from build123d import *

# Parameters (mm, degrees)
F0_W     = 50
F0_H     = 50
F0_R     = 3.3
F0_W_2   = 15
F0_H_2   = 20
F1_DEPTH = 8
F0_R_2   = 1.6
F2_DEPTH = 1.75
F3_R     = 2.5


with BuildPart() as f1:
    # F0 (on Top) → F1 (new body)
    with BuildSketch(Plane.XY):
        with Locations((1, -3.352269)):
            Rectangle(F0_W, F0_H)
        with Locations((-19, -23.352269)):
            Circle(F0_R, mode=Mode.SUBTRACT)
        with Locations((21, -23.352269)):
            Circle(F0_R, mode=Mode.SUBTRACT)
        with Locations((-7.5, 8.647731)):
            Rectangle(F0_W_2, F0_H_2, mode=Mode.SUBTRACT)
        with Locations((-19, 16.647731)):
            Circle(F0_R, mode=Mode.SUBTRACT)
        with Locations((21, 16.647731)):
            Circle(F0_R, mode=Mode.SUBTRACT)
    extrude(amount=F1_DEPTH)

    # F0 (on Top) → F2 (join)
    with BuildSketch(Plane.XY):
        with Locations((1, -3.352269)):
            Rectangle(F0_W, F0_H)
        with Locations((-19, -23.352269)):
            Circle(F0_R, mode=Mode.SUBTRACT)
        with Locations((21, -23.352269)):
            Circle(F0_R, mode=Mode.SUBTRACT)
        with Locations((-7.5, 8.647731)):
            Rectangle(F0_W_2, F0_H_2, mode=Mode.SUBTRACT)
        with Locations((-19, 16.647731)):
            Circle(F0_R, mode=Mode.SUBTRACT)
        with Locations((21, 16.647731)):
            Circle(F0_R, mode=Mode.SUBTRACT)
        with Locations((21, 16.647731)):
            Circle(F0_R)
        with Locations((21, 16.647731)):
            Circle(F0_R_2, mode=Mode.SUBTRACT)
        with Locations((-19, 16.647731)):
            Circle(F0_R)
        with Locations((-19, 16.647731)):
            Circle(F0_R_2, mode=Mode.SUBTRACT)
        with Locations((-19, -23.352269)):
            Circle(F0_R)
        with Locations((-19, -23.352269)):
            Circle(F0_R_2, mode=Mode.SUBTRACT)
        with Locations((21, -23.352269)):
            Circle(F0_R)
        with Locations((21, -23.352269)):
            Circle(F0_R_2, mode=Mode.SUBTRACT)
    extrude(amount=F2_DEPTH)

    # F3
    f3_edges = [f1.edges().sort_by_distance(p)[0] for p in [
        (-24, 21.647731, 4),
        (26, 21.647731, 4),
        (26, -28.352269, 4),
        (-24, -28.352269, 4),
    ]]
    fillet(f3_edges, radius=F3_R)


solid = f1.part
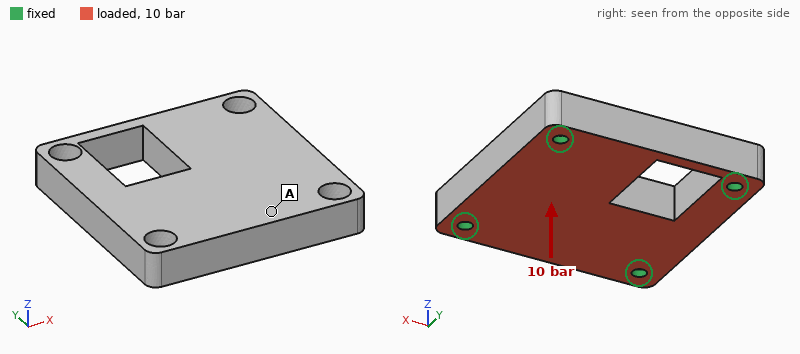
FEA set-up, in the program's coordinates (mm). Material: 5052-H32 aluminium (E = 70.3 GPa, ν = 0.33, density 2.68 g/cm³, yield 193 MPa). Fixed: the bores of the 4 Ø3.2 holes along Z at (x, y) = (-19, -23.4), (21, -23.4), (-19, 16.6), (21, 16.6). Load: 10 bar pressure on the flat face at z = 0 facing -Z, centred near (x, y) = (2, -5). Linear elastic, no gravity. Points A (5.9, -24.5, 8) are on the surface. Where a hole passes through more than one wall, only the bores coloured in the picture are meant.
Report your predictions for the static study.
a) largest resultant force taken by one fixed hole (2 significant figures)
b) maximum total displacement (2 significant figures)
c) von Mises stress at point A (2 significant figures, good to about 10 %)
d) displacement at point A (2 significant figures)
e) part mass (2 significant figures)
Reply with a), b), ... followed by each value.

a) 790 N
b) 20 µm
c) 14 MPa
d) 10 µm
e) 45 g
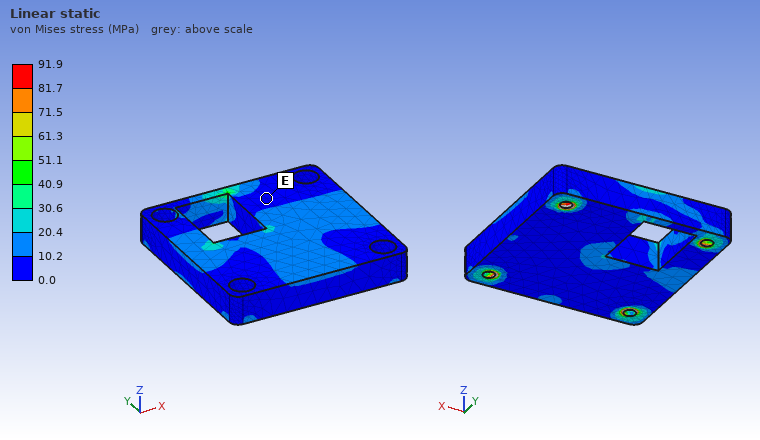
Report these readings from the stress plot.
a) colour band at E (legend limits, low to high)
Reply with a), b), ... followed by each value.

a) 0.0 to 10.2 MPa
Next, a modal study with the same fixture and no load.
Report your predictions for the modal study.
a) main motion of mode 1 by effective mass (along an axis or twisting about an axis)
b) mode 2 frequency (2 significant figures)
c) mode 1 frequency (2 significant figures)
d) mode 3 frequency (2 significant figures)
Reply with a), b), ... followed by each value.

a) along Z
b) 15 kHz
c) 9600 Hz
d) 15 kHz
